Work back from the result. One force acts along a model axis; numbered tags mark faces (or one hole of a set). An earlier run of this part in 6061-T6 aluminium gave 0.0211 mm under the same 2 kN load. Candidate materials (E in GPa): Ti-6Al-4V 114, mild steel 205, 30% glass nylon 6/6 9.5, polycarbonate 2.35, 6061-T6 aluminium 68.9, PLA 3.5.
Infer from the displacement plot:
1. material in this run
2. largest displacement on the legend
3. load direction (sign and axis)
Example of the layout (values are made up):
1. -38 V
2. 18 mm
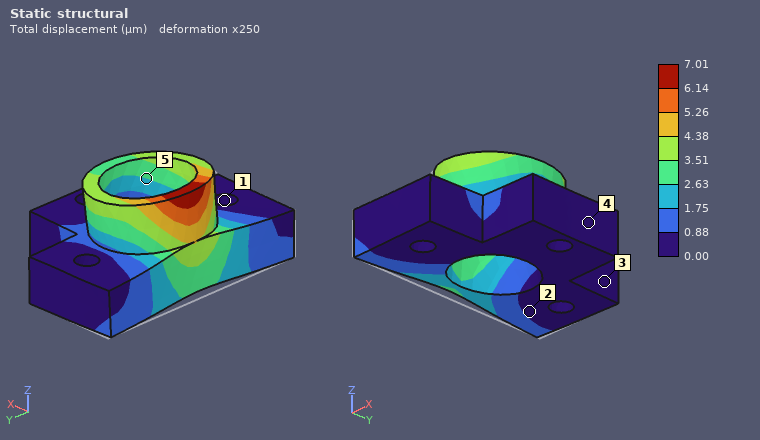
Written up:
1. mild steel
2. 7.01 µm
3. +X
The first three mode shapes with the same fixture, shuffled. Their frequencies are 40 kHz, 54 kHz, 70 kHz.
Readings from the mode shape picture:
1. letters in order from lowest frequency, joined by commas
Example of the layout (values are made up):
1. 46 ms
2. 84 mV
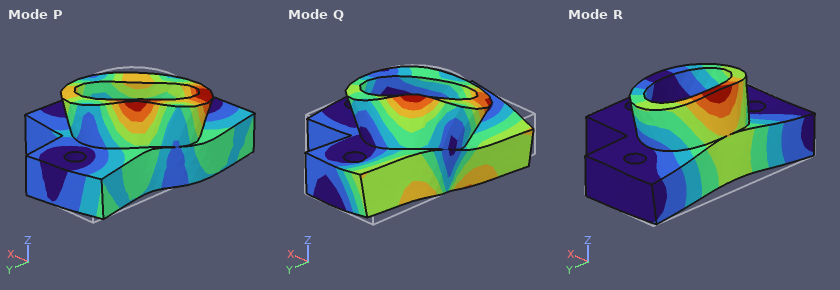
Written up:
1. R, P, Q
